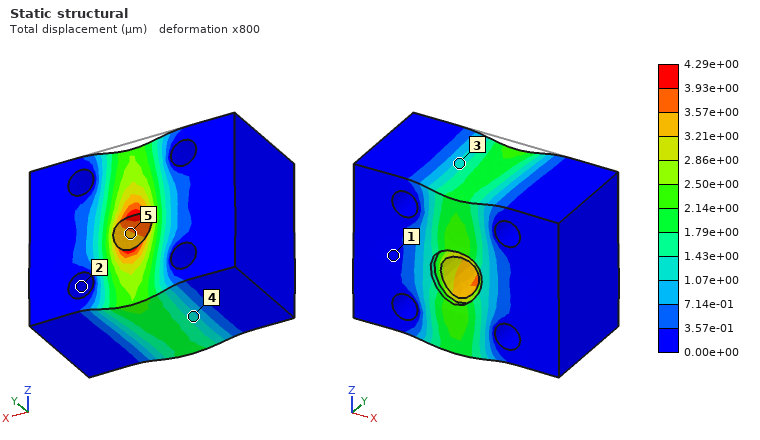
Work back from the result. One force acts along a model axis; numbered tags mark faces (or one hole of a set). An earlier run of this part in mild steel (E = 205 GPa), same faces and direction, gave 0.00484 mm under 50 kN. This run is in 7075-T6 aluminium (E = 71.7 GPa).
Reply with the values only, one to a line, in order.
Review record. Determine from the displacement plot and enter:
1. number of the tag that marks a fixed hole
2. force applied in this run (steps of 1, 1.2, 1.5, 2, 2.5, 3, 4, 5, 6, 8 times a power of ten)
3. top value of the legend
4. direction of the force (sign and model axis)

2
15 kN
4.29e+00 µm
-Z
